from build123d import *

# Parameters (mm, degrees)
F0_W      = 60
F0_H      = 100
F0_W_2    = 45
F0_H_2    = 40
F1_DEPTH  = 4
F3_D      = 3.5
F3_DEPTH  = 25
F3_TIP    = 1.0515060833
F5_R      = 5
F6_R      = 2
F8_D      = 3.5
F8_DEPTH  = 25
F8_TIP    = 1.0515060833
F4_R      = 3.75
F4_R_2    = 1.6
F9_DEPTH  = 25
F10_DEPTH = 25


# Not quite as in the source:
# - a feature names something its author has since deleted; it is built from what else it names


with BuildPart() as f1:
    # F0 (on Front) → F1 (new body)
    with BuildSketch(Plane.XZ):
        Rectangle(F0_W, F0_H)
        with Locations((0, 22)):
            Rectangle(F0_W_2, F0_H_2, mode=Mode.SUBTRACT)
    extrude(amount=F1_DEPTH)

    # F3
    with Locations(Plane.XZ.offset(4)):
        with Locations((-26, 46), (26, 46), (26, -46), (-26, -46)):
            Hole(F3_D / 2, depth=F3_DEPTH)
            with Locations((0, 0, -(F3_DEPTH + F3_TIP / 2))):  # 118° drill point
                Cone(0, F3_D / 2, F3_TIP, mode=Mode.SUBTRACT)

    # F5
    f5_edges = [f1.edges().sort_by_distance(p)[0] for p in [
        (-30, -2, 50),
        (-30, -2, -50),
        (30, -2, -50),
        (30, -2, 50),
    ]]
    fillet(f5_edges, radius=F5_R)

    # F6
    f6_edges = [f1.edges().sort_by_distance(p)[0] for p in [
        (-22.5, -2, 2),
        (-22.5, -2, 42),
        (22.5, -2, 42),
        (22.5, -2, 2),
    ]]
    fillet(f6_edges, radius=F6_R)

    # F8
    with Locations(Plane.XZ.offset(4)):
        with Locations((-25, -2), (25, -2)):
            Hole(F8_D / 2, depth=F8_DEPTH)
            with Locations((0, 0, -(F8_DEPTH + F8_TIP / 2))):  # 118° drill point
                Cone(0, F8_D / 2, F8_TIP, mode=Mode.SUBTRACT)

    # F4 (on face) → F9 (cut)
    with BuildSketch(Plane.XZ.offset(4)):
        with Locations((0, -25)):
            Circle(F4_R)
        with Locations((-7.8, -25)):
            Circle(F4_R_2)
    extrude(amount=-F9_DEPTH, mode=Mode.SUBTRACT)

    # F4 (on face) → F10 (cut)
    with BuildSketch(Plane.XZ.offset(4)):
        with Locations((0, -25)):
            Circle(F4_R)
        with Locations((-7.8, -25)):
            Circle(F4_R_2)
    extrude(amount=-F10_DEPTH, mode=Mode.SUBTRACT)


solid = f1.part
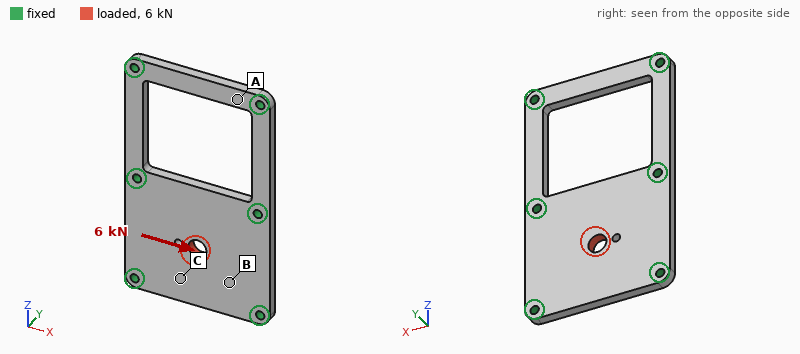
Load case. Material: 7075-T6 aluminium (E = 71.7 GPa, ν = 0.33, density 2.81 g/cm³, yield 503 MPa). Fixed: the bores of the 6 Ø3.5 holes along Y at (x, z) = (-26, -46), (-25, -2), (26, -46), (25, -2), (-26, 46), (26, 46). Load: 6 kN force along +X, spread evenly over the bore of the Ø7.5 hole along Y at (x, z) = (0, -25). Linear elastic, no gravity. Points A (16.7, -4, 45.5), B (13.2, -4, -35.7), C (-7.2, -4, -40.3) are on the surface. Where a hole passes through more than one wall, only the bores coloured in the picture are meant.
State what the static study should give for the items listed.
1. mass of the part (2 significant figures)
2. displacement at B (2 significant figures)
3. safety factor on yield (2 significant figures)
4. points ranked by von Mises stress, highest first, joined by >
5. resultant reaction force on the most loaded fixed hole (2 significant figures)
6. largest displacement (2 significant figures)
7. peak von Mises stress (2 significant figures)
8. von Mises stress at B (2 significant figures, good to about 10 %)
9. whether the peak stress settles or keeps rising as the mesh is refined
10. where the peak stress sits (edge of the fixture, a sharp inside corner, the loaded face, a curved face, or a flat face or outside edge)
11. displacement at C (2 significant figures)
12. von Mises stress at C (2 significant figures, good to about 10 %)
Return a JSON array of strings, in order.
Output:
["46 g", "9.2 µm", "3.4", "B > C > A", "1.7 kN", "21 µm", "150 MPa", "30 MPa", "settles", "a curved face", "7.5 µm", "19 MPa"]
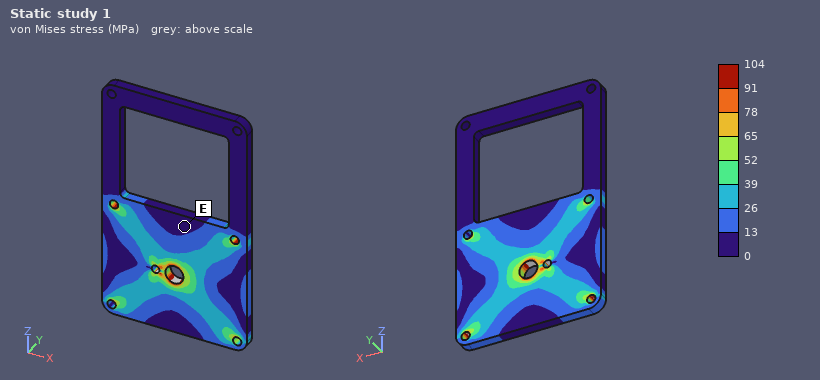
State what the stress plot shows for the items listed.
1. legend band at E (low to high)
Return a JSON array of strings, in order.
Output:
["0 to 13 MPa"]
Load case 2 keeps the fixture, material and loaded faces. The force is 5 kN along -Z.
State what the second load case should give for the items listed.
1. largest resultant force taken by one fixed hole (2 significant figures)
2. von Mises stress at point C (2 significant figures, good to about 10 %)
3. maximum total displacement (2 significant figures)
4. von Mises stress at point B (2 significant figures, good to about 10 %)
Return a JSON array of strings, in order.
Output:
["1.5 kN", "20 MPa", "19 µm", "27 MPa"]
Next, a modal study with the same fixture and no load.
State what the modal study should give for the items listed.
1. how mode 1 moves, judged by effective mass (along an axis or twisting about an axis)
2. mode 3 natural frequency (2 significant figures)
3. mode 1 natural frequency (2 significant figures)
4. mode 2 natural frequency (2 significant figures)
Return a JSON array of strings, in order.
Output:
["along Y", "9100 Hz", "5800 Hz", "8100 Hz"]
